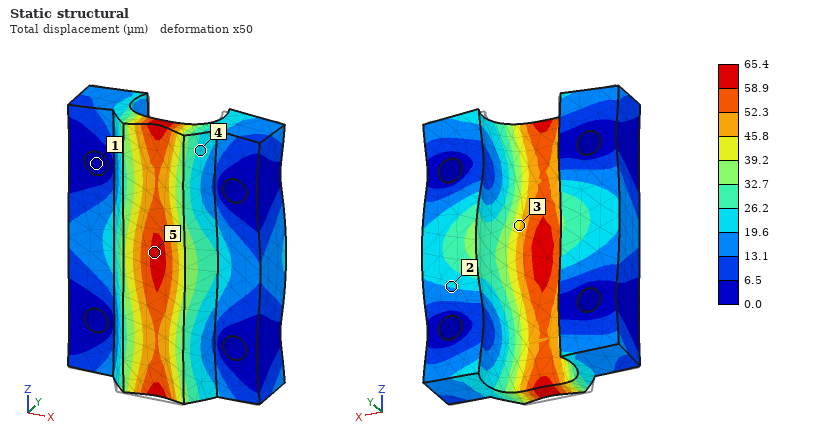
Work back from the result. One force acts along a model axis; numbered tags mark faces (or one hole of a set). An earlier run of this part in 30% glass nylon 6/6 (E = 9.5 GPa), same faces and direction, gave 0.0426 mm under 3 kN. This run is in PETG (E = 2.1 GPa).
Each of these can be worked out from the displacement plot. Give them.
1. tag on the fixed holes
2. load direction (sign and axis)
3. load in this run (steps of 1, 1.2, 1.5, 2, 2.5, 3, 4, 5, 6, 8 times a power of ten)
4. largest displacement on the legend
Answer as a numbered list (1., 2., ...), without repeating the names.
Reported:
1. 1
2. +Y
3. 1 kN
4. 65.4 µm
